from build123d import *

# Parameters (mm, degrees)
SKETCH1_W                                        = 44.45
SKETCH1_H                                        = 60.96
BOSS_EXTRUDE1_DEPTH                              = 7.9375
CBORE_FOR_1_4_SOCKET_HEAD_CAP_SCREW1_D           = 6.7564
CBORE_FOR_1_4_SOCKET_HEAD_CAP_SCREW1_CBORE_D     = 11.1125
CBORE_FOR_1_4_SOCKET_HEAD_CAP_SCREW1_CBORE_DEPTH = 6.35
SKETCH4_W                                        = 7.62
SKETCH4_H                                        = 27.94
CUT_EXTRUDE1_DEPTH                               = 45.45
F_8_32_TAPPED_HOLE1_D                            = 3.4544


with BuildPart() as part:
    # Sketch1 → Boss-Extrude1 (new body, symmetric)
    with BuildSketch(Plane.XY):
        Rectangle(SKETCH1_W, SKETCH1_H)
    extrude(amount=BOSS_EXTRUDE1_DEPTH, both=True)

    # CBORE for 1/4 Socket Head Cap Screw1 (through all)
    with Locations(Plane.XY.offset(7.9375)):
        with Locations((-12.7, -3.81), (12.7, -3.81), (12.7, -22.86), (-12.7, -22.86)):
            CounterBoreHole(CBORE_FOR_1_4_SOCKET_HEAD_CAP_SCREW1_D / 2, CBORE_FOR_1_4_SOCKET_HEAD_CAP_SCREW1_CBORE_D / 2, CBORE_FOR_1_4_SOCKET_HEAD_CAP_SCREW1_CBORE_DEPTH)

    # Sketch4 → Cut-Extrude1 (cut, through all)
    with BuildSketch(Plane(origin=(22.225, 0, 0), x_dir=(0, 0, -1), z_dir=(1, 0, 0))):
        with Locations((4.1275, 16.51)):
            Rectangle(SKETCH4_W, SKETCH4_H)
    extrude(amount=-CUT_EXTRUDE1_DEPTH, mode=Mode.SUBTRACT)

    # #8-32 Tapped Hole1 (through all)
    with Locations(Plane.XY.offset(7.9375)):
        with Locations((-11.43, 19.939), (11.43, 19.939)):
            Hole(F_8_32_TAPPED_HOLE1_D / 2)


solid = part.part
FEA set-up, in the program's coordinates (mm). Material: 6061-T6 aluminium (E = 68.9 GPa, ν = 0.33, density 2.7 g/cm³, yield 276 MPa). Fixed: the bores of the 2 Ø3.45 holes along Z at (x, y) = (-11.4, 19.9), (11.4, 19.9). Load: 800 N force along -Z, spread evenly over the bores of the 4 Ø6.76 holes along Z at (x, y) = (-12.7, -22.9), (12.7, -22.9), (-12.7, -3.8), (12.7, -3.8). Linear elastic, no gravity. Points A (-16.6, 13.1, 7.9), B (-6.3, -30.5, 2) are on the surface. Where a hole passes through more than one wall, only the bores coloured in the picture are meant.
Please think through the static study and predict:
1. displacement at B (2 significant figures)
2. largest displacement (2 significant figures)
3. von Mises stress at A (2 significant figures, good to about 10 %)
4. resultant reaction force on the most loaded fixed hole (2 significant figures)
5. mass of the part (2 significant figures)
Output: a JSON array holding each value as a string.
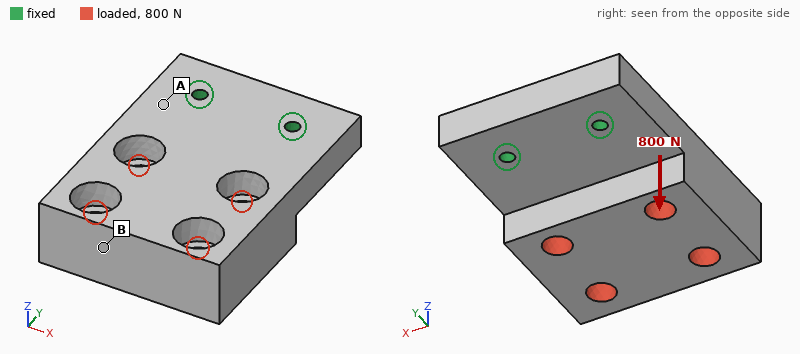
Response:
["0.14 mm", "0.15 mm", "38 MPa", "400 N", "80 g"]
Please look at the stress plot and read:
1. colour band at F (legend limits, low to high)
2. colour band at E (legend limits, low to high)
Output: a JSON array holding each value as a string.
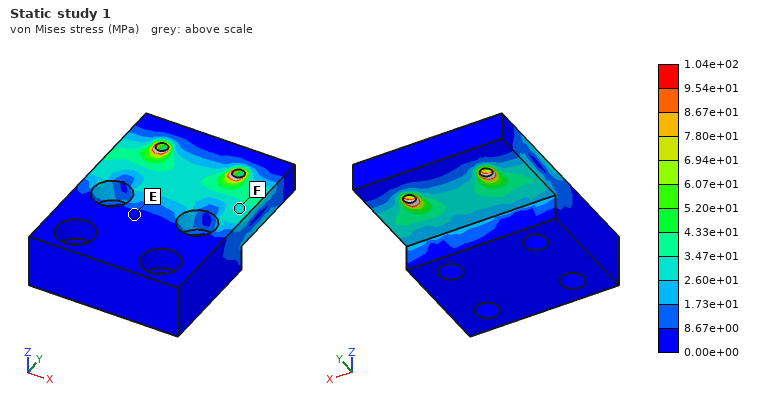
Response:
["2.60e+01 to 3.47e+01 MPa", "0.00e+00 to 8.67e+00 MPa"]
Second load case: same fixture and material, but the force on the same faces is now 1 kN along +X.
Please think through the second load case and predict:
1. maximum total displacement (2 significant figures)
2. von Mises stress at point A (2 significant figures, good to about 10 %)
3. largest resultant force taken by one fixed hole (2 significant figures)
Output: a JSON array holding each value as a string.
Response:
["20 µm", "9.2 MPa", "1.4 kN"]
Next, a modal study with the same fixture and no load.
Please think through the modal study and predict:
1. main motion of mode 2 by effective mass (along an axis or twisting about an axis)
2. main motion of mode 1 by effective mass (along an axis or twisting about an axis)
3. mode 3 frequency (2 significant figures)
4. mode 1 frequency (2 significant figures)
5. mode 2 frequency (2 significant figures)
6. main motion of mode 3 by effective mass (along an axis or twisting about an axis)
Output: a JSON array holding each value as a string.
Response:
["along X", "along Z", "6200 Hz", "1900 Hz", "5800 Hz", "along X"]
